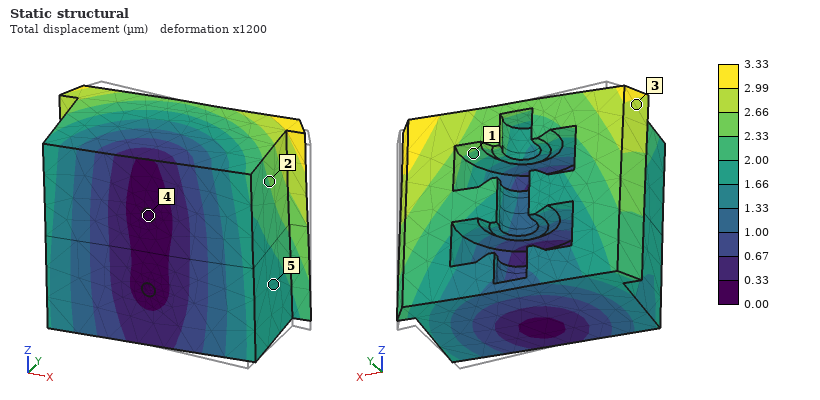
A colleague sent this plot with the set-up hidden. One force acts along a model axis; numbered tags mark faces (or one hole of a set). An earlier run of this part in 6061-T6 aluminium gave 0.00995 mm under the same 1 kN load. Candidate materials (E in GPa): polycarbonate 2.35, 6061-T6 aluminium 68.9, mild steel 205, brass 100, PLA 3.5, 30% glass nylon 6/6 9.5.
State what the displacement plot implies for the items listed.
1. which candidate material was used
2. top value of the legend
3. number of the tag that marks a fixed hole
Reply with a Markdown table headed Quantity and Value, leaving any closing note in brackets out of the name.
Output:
| Quantity | Value |
|---|---|
| which candidate material was used | mild steel |
| top value of the legend | 3.33 µm |
| number of the tag that marks a fixed hole | 4 |
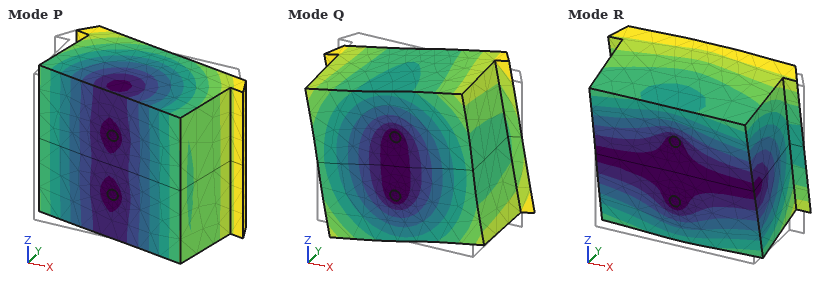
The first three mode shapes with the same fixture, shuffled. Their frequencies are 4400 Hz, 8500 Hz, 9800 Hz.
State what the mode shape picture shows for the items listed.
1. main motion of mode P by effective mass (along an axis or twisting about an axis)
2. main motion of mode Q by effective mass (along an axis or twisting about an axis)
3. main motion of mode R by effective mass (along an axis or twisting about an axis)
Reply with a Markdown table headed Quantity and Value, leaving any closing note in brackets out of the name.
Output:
| Quantity | Value |
|---|---|
| main motion of mode P by effective mass | along X |
| main motion of mode Q by effective mass | twisting about Y |
| main motion of mode R by effective mass | along Z |
